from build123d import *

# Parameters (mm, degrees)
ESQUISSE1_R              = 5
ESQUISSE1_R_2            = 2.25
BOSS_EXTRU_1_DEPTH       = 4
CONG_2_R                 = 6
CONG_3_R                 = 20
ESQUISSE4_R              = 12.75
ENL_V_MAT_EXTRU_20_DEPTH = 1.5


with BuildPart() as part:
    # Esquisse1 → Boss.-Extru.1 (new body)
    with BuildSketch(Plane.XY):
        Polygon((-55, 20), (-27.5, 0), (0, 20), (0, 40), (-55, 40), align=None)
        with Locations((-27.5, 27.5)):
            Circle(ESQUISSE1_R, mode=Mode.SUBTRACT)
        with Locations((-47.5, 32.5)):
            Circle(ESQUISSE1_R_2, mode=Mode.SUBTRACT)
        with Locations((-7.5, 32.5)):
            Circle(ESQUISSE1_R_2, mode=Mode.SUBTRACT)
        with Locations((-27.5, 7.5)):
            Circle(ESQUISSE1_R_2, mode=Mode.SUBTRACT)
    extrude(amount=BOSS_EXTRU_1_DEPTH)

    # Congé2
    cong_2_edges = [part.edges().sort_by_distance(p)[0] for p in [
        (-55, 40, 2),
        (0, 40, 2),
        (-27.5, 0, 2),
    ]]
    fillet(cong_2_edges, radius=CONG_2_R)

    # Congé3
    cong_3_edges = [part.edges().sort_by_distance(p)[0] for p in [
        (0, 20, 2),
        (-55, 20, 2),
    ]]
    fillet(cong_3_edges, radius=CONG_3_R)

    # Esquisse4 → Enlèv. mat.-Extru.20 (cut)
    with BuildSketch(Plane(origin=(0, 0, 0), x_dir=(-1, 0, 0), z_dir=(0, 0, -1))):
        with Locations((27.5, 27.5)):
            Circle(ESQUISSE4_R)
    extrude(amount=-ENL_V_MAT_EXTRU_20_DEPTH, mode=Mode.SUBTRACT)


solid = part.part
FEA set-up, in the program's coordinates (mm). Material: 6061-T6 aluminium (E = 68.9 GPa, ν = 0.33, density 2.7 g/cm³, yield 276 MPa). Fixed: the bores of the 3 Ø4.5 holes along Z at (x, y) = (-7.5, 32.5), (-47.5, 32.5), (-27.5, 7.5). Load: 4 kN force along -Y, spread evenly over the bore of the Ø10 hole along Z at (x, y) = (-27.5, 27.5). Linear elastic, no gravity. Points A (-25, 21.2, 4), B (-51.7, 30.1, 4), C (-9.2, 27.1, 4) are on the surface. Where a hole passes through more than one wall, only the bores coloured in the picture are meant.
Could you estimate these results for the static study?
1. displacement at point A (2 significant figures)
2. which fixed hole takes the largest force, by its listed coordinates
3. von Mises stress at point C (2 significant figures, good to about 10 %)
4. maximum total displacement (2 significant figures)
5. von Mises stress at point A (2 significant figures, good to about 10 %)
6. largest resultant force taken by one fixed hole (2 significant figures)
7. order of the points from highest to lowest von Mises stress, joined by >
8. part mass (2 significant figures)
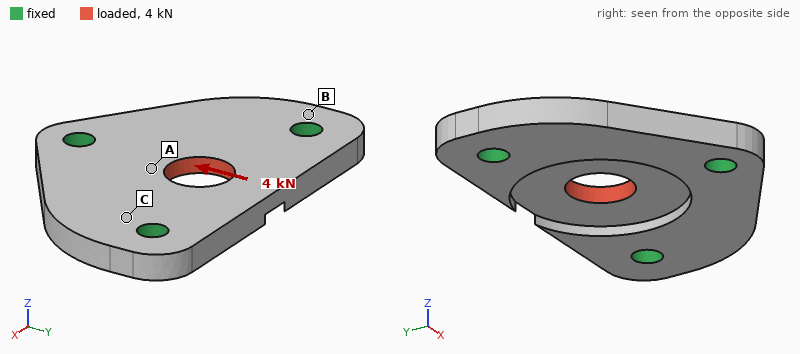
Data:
12 µm
(-27.5, 7.5)
30 MPa
26 µm
69 MPa
1.8 kN
A > C > B
14 g
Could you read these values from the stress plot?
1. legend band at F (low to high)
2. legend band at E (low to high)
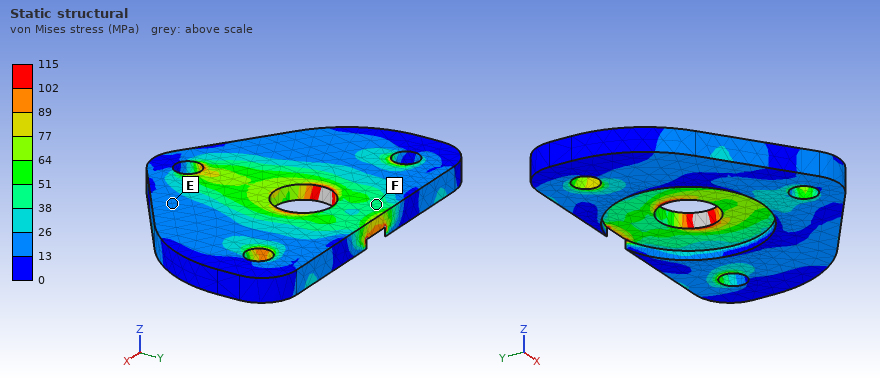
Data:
38 to 51 MPa
13 to 26 MPa
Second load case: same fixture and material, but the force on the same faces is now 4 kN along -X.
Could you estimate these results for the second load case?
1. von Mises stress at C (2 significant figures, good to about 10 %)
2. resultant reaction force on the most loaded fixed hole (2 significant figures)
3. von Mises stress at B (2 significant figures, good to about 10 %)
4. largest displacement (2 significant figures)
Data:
28 MPa
1.5 kN
12 MPa
13 µm
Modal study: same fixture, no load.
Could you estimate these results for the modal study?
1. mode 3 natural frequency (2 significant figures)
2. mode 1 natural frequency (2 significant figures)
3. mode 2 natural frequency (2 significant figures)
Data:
17 kHz
15 kHz
17 kHz
